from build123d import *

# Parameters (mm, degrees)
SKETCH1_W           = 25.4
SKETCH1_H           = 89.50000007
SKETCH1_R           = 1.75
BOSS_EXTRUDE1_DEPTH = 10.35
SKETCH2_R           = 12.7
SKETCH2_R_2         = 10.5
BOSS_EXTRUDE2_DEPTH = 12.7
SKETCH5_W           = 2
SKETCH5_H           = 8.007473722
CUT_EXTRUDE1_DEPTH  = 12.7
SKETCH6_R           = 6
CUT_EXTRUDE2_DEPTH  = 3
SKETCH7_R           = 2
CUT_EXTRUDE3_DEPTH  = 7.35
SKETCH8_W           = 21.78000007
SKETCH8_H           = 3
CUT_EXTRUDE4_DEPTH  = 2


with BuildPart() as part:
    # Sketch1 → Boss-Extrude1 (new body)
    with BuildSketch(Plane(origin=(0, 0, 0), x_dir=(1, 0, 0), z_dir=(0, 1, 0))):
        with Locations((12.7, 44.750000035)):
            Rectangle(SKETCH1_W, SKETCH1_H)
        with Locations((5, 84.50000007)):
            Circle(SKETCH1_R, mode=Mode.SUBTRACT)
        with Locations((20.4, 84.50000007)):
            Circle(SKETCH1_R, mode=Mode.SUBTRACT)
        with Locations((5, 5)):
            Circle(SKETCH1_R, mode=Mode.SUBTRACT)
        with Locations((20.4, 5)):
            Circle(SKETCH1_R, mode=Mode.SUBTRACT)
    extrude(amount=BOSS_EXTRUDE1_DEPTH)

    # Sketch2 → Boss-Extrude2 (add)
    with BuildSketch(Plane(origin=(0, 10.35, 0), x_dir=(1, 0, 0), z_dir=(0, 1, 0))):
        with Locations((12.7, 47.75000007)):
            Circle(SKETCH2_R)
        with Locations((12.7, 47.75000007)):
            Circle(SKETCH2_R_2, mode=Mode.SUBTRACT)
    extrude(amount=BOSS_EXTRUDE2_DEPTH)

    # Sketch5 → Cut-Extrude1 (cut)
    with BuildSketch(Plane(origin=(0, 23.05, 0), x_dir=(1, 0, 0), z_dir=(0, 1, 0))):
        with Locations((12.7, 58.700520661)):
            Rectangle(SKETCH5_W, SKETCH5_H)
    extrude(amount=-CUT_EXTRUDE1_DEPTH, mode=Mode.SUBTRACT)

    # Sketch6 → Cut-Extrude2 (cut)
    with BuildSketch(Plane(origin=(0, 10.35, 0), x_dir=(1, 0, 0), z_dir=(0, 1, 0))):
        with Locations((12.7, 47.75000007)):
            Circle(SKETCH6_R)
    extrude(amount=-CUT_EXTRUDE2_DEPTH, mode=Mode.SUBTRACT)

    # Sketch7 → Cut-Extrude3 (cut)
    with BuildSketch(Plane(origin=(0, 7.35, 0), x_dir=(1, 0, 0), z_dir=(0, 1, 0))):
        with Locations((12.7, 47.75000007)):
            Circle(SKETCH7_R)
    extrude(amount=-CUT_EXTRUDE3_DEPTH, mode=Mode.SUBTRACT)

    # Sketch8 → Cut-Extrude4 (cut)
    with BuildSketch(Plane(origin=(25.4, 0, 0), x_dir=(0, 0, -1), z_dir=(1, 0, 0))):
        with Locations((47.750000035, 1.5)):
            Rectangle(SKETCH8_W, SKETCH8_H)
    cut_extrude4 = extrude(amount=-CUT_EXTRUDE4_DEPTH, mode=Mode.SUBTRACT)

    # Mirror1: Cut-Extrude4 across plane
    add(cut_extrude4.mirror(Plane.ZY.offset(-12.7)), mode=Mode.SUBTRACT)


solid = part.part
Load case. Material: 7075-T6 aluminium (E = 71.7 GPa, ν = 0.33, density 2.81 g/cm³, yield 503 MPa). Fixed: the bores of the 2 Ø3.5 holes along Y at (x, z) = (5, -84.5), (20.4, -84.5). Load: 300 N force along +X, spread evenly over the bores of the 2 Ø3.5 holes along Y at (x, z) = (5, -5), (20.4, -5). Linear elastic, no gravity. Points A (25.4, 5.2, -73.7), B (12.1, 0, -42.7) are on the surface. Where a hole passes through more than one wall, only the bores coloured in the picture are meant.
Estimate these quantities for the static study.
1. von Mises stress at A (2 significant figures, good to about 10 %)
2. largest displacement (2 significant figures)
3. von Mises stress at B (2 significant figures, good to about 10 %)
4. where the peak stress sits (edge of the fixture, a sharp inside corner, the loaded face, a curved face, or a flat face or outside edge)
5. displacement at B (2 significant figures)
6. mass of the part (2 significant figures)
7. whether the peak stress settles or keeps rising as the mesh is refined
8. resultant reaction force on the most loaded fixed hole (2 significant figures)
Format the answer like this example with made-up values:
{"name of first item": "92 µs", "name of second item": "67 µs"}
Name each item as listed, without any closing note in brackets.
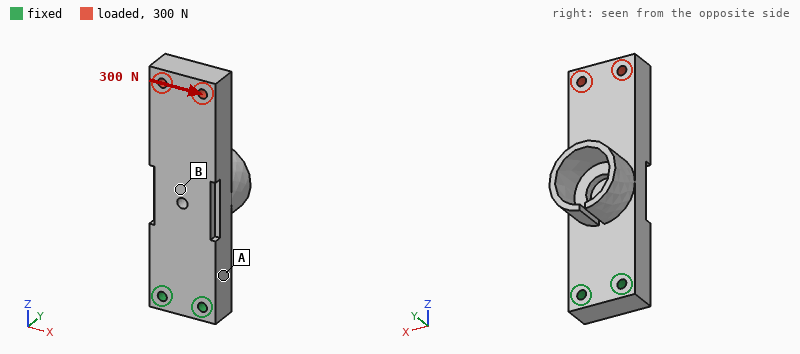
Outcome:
{"von Mises stress at A": "18 MPa", "largest displacement": "63 µm", "von Mises stress at B": "3.8 MPa", "where the peak stress sits": "edge of the fixture", "displacement at B": "20 µm", "mass of the part": "69 g", "whether the peak stress settles or keeps rising as the mesh is refined": "keeps rising", "resultant reaction force on the most loaded fixed hole": "1.4 kN"}
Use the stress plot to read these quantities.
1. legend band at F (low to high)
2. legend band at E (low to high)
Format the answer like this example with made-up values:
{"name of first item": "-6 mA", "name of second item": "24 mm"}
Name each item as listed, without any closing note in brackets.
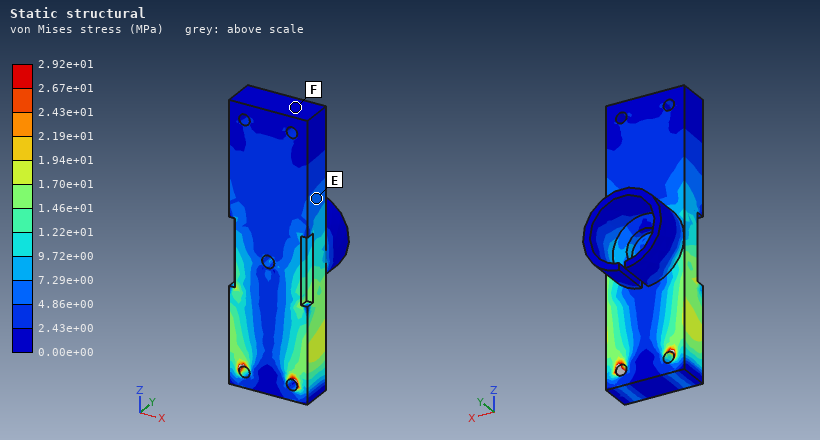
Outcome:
{"legend band at F": "0.00e+00 to 2.43e+00 MPa", "legend band at E": "4.86e+00 to 7.29e+00 MPa"}
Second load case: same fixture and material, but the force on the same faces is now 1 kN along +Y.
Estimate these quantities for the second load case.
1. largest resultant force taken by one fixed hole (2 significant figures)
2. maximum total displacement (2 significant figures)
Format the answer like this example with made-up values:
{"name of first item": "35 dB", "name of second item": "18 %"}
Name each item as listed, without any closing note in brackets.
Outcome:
{"largest resultant force taken by one fixed hole": "500 N", "maximum total displacement": "1.1 mm"}
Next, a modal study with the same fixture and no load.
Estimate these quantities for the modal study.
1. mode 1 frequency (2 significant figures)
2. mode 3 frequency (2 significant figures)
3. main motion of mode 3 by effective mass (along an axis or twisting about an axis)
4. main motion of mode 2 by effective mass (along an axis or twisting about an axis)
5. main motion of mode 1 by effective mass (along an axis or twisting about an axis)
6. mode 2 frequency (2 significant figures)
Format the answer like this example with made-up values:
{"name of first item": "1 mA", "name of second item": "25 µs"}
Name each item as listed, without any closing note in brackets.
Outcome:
{"mode 1 frequency": "1100 Hz", "mode 3 frequency": "5600 Hz", "main motion of mode 3 by effective mass": "twisting about Z", "main motion of mode 2 by effective mass": "along X", "main motion of mode 1 by effective mass": "along Y", "mode 2 frequency": "2600 Hz"}
